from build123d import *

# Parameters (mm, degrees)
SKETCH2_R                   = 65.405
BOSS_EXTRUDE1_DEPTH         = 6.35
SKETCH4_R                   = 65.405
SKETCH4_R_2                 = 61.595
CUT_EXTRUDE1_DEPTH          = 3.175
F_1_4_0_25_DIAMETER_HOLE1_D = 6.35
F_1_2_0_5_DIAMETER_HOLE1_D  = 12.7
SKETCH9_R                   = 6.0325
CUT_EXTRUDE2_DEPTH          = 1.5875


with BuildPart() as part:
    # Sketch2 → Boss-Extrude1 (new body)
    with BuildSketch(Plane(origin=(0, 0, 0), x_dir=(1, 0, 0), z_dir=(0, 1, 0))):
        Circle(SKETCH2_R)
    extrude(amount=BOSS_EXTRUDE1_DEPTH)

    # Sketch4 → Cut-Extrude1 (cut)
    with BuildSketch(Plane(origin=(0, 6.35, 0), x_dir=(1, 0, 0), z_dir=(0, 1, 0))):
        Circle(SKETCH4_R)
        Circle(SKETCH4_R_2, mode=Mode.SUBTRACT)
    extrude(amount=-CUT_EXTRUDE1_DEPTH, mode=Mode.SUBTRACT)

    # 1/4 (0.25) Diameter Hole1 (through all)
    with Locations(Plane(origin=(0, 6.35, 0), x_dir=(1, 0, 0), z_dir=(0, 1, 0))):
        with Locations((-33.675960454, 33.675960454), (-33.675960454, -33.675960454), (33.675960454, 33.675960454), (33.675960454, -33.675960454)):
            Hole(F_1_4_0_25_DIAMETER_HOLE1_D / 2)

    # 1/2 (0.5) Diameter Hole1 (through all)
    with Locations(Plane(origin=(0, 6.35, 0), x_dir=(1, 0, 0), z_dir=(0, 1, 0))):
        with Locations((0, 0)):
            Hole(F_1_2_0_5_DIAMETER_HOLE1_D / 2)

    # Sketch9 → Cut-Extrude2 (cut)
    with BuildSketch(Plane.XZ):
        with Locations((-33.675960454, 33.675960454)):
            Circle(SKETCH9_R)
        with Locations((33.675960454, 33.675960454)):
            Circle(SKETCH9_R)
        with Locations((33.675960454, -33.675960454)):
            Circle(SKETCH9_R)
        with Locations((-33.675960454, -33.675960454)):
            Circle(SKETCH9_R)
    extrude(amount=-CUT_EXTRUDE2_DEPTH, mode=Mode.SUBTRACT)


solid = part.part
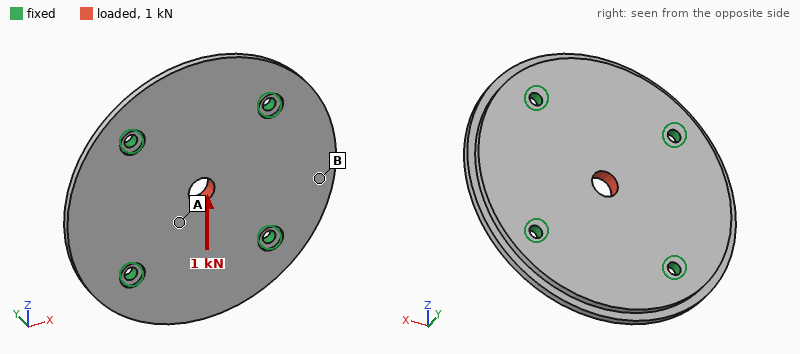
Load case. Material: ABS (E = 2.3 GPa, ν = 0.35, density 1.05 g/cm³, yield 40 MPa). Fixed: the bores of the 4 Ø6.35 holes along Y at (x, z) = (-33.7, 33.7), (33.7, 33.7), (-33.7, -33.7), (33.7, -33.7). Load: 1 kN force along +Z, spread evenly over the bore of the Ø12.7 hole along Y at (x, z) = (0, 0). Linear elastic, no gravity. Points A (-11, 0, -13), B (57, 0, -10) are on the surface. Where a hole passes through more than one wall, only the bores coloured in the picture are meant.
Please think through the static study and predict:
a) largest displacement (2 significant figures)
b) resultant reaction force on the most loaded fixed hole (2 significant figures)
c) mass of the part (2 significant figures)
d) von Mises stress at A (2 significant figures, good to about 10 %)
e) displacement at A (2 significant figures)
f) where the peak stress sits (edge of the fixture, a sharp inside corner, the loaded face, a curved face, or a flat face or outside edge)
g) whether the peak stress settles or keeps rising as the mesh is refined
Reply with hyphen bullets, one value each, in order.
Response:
- 51 µm
- 260 N
- 82 g
- 2.2 MPa
- 32 µm
- edge of the fixture
- keeps rising
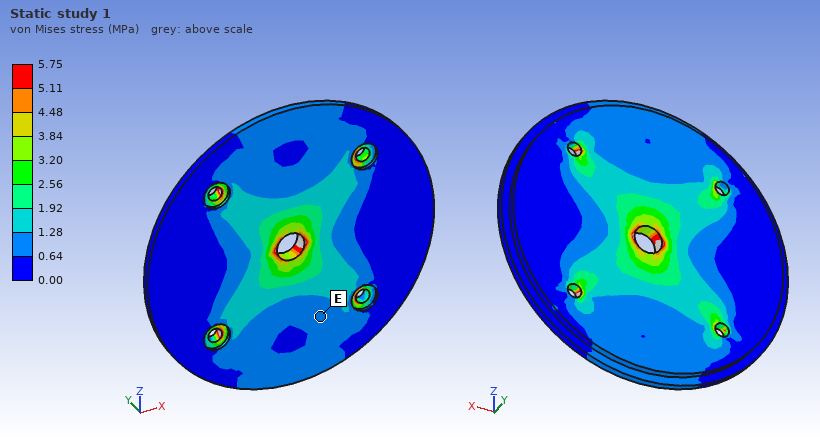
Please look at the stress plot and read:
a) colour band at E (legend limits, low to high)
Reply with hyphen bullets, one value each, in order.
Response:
- 0.64 to 1.28 MPa
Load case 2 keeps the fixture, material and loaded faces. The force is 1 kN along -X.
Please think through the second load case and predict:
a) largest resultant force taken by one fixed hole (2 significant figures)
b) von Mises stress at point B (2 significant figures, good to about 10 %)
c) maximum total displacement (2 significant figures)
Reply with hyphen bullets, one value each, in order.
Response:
- 260 N
- 0.74 MPa
- 51 µm
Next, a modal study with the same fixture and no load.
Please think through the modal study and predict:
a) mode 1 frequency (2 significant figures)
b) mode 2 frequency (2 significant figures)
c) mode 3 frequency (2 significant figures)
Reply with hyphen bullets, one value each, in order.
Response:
- 1100 Hz
- 1200 Hz
- 1200 Hz
